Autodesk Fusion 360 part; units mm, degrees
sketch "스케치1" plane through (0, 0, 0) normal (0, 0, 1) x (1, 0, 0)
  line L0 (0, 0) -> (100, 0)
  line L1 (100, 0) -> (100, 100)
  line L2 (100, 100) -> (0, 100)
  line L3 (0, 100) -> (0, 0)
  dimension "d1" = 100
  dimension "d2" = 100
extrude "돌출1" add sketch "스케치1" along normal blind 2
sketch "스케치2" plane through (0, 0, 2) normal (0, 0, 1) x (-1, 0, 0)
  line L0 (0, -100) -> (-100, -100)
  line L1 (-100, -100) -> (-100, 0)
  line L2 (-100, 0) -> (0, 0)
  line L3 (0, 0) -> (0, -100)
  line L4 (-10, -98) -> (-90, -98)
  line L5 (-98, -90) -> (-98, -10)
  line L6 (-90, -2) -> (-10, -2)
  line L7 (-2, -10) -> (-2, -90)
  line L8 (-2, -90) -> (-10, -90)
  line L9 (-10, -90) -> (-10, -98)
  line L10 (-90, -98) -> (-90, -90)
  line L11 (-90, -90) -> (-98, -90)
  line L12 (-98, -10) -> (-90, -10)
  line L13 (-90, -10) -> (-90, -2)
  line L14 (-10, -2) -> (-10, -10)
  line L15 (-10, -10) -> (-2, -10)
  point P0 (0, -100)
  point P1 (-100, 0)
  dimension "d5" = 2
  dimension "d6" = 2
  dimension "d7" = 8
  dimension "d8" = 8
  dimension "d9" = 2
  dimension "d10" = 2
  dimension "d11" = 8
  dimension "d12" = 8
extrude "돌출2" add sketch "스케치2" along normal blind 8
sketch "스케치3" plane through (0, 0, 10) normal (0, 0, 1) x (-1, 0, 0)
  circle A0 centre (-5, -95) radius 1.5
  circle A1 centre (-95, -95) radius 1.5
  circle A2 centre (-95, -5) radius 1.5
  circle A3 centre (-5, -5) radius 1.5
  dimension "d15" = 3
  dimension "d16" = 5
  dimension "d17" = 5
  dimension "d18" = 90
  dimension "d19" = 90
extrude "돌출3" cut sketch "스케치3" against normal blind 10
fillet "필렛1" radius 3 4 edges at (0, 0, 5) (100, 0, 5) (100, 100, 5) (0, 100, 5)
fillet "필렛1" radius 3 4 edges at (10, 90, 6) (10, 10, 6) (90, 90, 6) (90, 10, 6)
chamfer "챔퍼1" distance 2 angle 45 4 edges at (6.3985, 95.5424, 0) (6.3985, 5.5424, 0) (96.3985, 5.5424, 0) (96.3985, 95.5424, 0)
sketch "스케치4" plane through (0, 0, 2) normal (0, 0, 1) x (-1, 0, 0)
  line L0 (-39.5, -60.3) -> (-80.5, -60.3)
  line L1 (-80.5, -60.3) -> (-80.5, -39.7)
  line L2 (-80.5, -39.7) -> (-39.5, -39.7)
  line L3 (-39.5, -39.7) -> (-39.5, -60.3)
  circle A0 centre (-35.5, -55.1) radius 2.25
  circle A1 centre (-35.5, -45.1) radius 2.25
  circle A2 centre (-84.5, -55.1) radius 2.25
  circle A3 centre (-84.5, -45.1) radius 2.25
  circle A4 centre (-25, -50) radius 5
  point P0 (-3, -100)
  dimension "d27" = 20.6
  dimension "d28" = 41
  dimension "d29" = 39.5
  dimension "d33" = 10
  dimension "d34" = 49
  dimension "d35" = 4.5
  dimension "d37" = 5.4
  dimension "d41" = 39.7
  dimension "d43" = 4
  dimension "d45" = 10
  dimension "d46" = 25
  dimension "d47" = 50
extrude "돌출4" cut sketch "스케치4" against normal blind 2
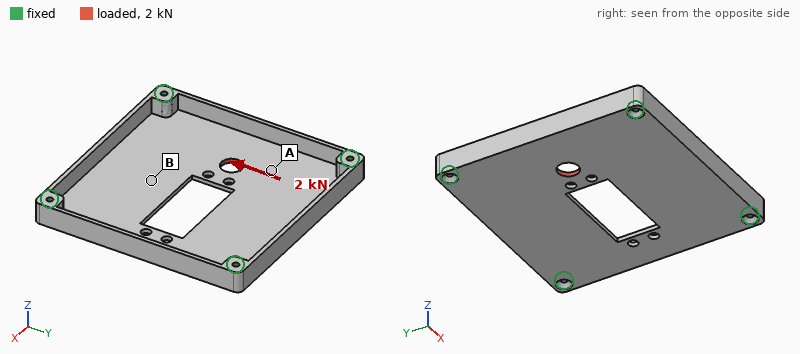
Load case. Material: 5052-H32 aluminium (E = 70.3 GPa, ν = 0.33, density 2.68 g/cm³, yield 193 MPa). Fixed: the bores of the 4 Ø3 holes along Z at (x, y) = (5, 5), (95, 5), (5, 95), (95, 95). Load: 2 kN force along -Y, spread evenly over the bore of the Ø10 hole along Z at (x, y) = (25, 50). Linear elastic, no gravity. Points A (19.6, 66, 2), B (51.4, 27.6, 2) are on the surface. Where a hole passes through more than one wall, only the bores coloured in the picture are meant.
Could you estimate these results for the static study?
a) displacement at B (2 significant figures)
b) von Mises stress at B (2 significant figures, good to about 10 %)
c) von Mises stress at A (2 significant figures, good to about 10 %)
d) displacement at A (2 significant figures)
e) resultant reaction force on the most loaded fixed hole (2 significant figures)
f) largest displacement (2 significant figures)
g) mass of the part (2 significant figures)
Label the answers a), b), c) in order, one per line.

a) 9.2 µm
b) 5.9 MPa
c) 20 MPa
d) 11 µm
e) 860 N
f) 17 µm
g) 69 g
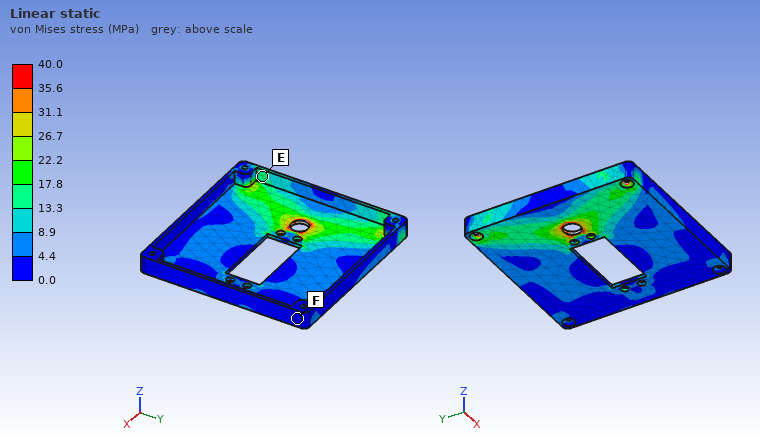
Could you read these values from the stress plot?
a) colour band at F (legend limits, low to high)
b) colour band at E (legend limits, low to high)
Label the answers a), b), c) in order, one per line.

a) 0.0 to 4.4 MPa
b) 13.3 to 17.8 MPa
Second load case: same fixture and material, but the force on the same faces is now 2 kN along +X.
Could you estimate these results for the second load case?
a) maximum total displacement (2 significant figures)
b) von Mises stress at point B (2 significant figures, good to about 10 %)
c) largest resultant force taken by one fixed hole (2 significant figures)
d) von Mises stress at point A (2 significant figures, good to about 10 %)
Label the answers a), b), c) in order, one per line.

a) 29 µm
b) 14 MPa
c) 570 N
d) 22 MPa
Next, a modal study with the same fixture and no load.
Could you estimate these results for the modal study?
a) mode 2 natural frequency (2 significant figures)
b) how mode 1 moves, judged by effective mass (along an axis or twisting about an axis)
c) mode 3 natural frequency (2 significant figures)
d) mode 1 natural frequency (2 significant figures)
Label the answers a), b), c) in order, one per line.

a) 2200 Hz
b) along Z
c) 2700 Hz
d) 1300 Hz
